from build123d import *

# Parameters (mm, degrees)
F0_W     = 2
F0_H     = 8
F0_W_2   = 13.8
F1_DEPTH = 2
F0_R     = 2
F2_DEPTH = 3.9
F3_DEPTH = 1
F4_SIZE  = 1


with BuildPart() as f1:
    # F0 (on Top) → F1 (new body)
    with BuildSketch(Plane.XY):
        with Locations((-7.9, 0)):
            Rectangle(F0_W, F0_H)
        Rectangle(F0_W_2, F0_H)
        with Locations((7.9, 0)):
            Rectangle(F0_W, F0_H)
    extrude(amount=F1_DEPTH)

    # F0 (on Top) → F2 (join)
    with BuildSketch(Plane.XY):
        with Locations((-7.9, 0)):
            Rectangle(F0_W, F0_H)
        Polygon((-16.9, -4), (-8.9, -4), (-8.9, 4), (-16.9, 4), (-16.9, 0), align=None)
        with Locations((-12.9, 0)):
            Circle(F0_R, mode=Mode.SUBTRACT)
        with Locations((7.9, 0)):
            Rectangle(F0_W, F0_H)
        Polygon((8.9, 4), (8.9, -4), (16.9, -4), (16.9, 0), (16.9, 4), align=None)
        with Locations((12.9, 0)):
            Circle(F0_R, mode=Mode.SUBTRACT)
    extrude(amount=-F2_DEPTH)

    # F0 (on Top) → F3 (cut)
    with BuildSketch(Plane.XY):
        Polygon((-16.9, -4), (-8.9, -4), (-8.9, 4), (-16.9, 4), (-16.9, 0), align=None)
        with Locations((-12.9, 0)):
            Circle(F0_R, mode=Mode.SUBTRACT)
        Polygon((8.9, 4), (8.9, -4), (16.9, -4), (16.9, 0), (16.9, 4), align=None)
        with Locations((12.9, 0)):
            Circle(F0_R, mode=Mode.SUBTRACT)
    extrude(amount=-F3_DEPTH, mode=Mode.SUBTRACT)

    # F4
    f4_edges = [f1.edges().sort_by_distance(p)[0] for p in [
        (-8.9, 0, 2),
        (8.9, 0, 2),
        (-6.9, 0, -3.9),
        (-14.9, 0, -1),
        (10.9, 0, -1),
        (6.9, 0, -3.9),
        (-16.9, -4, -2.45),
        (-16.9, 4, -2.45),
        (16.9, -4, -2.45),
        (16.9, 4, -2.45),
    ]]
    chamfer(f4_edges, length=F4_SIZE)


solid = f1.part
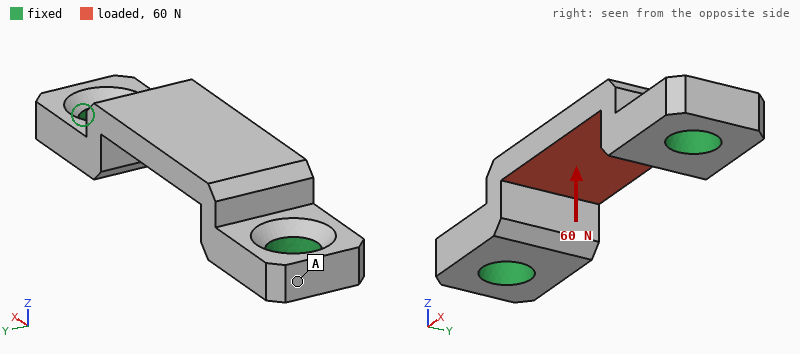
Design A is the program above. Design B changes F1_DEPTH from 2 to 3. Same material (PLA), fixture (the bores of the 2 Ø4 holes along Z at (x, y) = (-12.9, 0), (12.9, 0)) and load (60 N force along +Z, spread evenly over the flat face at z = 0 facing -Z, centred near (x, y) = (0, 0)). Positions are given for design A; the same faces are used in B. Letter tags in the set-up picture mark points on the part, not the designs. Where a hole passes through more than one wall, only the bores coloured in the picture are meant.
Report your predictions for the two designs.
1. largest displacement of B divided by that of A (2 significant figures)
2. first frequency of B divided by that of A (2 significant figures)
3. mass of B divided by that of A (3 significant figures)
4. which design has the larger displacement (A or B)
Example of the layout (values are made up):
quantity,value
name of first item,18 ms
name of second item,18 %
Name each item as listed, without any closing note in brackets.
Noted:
quantity,value
largest displacement of B divided by that of A,0.50
first frequency of B divided by that of A,0.79
mass of B divided by that of A,1.21
which design has the larger displacement,A
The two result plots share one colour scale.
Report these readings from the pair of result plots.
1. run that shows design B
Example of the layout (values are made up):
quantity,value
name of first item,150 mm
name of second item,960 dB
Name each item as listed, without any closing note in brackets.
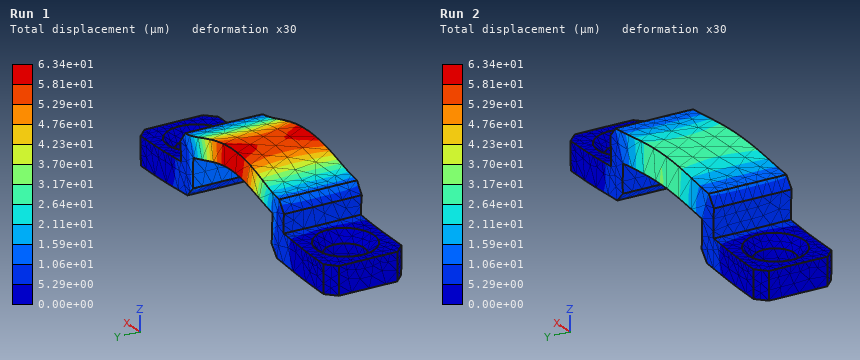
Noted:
quantity,value
run that shows design B,Run 2
